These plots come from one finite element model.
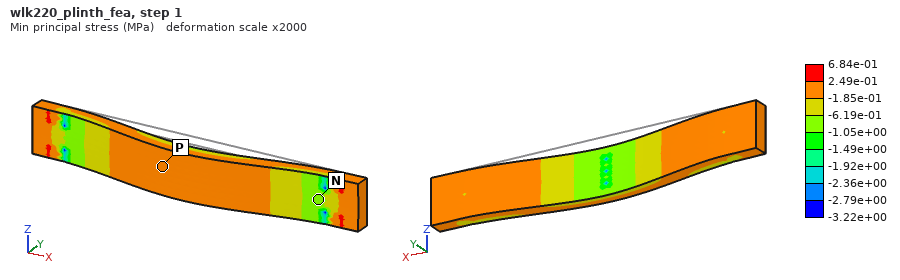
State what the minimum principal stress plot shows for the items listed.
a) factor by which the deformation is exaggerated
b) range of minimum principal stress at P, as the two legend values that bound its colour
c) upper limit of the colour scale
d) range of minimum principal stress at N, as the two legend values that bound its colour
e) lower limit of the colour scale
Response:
2000
-1.85e-01 to 2.49e-01 MPa
6.84e-01 MPa
-1.05e+00 to -6.19e-01 MPa
-3.22e+00 MPa
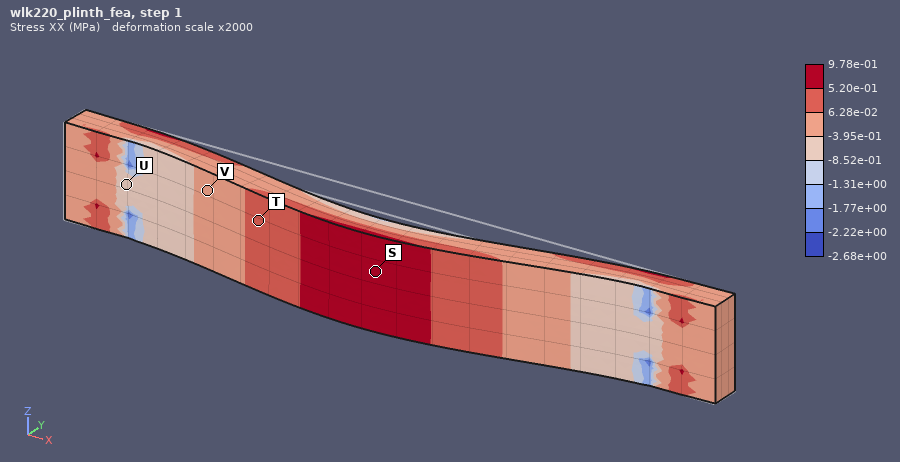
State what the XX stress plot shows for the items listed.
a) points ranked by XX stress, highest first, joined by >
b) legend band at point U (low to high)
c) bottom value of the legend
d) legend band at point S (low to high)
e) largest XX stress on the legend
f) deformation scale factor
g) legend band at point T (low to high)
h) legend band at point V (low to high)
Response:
S > T > V > U
-8.52e-01 to -3.95e-01 MPa
-2.68e+00 MPa
5.20e-01 to 9.78e-01 MPa
9.78e-01 MPa
2000
6.28e-02 to 5.20e-01 MPa
-3.95e-01 to 6.28e-02 MPa
